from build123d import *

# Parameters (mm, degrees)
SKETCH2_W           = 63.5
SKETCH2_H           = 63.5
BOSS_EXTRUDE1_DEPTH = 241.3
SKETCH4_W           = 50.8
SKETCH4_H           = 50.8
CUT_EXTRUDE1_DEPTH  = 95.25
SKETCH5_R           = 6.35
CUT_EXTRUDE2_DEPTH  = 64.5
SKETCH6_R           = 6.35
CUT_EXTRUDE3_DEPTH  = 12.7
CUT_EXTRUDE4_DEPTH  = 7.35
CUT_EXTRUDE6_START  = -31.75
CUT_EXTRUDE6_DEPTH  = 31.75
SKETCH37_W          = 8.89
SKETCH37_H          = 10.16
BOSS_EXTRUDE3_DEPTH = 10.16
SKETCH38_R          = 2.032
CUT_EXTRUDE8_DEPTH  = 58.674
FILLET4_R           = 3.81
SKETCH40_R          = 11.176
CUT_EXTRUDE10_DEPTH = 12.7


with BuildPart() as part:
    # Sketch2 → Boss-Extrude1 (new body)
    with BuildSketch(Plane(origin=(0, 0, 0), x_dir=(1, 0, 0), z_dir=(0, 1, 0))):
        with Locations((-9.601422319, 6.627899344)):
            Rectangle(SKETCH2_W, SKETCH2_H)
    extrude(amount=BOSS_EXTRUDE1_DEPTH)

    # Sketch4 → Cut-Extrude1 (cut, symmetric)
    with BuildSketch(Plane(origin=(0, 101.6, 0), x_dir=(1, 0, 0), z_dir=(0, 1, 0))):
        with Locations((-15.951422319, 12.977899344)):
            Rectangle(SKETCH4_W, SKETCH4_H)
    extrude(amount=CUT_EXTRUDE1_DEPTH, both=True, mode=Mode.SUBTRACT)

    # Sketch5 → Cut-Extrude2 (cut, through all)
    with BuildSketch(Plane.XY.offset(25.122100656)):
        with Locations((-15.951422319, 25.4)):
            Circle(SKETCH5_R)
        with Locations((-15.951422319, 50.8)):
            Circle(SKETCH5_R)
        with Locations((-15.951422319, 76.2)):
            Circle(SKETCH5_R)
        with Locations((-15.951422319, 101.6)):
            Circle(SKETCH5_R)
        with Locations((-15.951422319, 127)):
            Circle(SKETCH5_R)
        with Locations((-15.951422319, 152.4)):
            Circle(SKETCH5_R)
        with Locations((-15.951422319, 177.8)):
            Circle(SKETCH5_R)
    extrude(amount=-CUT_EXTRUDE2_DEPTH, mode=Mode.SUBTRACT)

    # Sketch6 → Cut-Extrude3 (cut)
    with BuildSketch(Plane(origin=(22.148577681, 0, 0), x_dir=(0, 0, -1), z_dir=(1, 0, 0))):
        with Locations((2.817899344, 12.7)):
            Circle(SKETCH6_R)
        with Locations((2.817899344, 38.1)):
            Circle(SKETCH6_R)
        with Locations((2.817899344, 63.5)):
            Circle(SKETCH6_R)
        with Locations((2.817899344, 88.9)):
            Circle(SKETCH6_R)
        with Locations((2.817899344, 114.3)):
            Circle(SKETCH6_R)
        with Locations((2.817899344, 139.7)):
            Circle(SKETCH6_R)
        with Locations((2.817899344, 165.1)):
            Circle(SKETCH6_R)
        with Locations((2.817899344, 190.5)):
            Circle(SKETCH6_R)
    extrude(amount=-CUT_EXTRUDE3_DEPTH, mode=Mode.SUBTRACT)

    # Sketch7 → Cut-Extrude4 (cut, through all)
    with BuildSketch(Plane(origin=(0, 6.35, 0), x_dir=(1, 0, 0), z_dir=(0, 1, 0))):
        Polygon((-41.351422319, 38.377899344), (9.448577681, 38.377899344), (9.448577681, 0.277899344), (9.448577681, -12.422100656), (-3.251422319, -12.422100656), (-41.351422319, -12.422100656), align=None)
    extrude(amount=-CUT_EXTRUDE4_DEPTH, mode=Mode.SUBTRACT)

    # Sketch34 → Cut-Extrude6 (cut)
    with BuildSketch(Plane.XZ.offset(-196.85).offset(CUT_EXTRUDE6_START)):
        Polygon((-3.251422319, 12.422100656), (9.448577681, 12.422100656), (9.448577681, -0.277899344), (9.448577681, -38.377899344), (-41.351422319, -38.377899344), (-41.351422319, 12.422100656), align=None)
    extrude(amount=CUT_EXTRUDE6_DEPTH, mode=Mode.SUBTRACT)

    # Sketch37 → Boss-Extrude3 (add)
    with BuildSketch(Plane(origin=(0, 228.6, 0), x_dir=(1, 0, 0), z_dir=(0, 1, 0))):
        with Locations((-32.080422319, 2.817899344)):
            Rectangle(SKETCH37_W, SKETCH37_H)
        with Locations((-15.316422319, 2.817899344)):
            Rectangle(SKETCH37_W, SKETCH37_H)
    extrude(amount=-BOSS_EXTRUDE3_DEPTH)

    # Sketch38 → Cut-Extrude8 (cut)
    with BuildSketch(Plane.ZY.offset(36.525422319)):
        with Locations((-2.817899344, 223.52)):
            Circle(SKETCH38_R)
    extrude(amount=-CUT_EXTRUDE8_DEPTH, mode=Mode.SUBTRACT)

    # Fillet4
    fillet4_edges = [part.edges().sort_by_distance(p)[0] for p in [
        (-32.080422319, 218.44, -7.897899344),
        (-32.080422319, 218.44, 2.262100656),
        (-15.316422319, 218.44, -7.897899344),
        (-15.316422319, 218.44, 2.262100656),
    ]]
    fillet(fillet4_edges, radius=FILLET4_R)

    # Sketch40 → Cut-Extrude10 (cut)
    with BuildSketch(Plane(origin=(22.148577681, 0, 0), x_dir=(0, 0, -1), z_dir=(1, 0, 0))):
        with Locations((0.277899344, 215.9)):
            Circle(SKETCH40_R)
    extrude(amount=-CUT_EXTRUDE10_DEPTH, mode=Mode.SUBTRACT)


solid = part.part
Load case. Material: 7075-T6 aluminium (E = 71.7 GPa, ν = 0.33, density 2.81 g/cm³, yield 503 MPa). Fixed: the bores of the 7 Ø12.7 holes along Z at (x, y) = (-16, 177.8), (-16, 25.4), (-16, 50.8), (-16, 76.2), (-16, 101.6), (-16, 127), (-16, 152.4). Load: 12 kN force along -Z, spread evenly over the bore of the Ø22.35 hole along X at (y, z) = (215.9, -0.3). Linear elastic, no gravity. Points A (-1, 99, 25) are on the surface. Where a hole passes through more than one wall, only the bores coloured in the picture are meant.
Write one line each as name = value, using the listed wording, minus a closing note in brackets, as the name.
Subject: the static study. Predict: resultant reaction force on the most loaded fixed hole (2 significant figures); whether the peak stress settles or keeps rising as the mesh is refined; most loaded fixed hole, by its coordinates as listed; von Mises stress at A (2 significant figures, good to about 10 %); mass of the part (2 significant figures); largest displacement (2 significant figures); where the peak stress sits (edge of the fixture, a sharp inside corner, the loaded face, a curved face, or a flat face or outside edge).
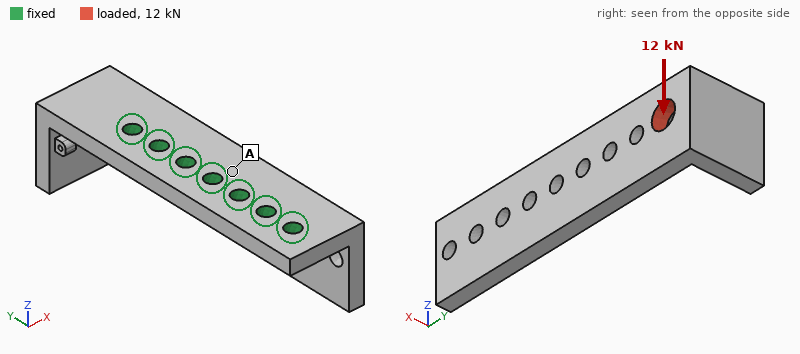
resultant reaction force on the most loaded fixed hole = 11 kN
whether the peak stress settles or keeps rising as the mesh is refined = keeps rising
most loaded fixed hole, by its coordinates as listed = (-16, 177.8)
von Mises stress at A = 24 MPa
mass of the part = 1000 g
largest displacement = 0.47 mm
where the peak stress sits = edge of the fixture
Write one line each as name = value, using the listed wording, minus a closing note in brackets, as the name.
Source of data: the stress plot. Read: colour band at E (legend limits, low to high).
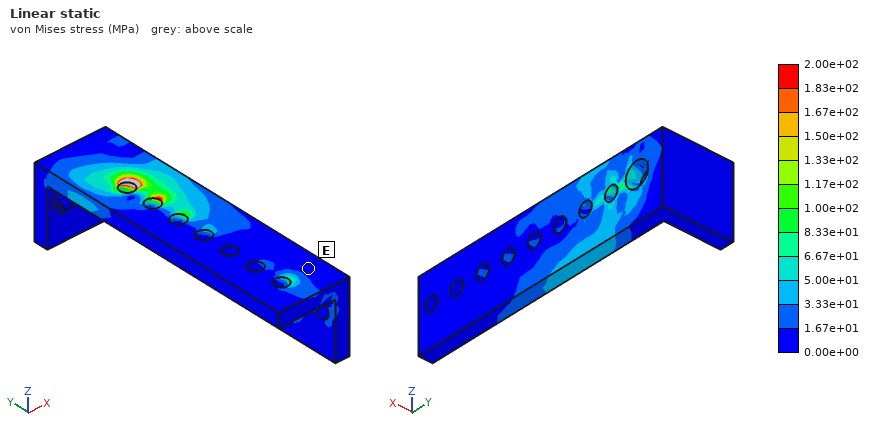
colour band at E = 0.00e+00 to 1.67e+01 MPa
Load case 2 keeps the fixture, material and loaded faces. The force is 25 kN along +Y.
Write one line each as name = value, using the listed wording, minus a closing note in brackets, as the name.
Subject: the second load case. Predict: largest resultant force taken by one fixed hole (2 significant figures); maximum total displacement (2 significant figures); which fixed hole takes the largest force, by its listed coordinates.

largest resultant force taken by one fixed hole = 12 kN
maximum total displacement = 0.11 mm
which fixed hole takes the largest force, by its listed coordinates = (-16, 177.8)
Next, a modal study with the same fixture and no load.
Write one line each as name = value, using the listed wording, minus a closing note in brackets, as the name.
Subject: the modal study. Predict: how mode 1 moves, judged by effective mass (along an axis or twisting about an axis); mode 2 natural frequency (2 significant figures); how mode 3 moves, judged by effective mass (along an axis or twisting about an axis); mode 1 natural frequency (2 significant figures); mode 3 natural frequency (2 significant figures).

how mode 1 moves, judged by effective mass = along X
mode 2 natural frequency = 2000 Hz
how mode 3 moves, judged by effective mass = along Z
mode 1 natural frequency = 1600 Hz
mode 3 natural frequency = 2300 Hz
